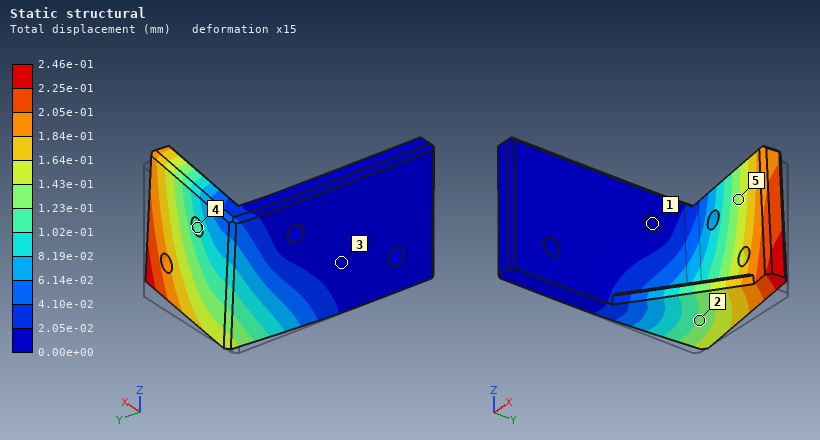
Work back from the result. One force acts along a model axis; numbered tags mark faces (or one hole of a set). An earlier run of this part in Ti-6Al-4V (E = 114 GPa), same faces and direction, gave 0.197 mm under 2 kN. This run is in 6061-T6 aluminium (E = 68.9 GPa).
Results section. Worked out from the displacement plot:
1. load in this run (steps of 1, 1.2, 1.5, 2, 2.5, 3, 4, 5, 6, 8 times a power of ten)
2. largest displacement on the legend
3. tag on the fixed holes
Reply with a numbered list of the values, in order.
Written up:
1. 1.5 kN
2. 2.46e-01 mm
3. 1
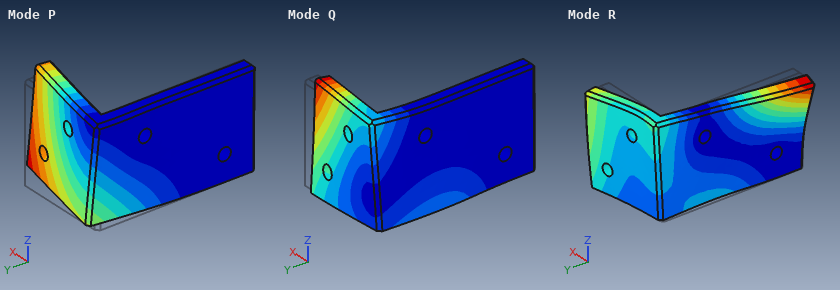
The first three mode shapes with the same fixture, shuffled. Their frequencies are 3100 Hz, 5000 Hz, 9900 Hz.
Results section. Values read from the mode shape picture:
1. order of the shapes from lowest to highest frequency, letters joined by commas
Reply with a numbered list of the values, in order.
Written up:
1. P, Q, R
